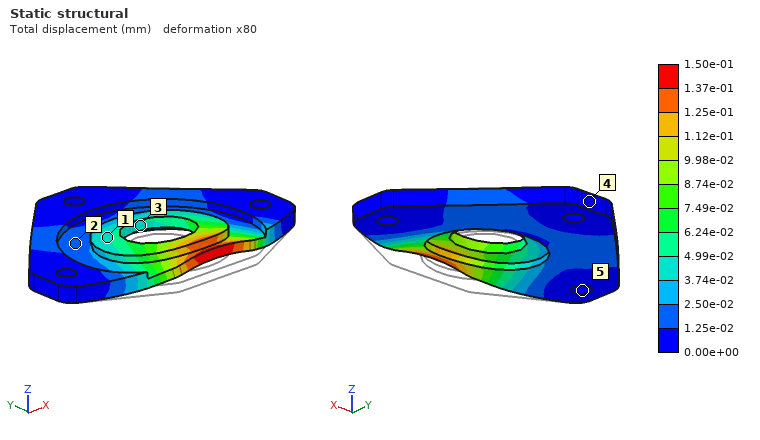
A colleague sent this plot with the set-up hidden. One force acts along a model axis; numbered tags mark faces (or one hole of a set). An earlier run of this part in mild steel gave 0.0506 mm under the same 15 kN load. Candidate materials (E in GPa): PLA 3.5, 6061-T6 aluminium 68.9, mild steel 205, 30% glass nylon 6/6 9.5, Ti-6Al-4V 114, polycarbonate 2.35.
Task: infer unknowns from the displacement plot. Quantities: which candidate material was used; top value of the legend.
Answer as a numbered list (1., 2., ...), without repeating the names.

1. 6061-T6 aluminium
2. 1.50e-01 mm
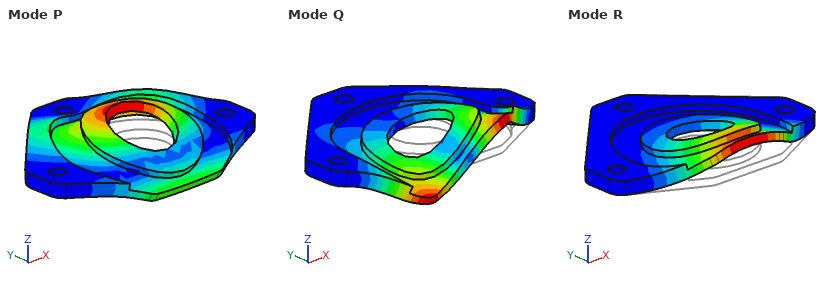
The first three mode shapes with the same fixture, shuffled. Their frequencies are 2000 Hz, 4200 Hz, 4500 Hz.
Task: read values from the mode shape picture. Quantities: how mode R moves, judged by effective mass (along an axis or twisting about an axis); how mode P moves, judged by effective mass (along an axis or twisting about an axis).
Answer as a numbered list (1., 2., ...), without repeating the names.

1. along Z
2. along Z
